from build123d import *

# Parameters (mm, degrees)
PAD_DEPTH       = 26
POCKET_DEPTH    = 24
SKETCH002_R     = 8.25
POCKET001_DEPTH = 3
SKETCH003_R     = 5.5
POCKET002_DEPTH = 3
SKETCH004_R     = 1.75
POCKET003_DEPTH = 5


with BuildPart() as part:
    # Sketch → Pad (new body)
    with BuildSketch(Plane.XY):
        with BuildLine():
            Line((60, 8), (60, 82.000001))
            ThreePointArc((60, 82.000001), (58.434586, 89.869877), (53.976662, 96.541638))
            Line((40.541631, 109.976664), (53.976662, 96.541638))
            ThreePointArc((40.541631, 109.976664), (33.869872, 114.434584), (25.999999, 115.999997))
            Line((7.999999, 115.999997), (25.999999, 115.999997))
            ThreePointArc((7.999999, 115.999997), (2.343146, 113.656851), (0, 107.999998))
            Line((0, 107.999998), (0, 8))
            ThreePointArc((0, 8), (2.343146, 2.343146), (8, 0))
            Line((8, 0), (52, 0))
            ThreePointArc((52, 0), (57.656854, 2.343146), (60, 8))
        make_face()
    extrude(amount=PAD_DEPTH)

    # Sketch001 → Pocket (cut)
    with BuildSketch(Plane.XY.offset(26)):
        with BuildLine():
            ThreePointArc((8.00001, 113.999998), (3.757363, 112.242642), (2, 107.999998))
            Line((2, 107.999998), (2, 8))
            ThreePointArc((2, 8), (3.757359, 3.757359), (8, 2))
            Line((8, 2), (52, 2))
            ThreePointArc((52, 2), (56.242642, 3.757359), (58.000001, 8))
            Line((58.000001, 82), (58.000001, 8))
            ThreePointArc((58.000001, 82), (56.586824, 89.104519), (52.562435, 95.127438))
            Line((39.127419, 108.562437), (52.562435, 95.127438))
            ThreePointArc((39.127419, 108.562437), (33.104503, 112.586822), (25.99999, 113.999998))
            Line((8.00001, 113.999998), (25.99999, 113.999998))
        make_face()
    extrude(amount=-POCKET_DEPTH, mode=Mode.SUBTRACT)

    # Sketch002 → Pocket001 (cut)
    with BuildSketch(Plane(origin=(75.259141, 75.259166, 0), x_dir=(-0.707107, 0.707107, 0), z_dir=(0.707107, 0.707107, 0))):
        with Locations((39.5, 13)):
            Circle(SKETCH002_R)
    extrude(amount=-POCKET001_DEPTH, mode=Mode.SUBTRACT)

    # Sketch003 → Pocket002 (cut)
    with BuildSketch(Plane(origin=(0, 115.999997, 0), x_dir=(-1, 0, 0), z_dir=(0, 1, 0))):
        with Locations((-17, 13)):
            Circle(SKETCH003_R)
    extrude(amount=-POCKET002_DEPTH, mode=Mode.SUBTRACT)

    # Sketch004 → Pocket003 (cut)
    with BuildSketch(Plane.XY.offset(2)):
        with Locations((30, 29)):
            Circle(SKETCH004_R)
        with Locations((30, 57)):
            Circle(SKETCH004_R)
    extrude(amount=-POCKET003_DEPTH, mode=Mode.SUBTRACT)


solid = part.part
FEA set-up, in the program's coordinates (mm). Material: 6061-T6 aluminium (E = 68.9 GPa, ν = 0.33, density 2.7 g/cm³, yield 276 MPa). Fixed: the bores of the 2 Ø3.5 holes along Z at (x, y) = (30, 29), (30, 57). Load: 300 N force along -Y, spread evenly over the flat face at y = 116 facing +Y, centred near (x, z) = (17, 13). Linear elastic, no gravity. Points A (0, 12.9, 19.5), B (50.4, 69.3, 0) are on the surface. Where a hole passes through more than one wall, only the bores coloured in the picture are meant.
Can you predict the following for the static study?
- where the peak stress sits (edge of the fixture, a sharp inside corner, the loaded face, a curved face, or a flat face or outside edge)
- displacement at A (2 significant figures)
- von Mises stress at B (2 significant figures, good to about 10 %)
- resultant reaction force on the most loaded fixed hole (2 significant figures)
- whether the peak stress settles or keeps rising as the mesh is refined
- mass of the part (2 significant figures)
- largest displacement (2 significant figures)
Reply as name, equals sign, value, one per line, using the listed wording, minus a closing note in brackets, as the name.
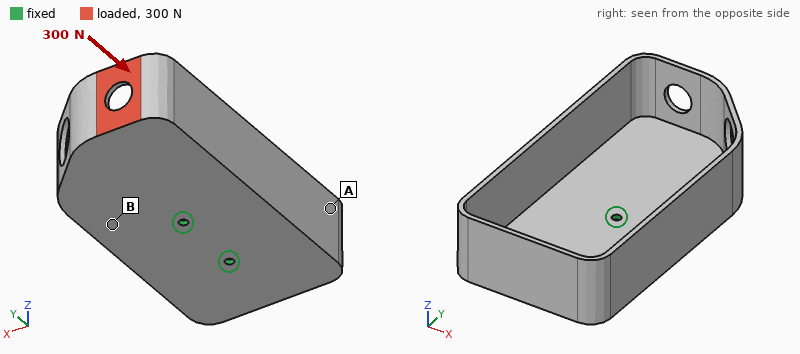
where the peak stress sits = edge of the fixture
displacement at A = 0.11 mm
von Mises stress at B = 12 MPa
resultant reaction force on the most loaded fixed hole = 230 N
whether the peak stress settles or keeps rising as the mesh is refined = keeps rising
mass of the part = 75 g
largest displacement = 0.31 mm
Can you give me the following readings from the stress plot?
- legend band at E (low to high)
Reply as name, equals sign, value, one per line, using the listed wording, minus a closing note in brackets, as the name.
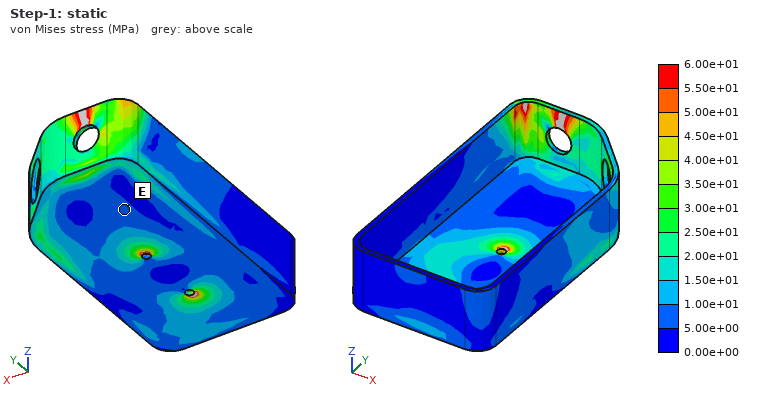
legend band at E = 5.00e+00 to 1.00e+01 MPa
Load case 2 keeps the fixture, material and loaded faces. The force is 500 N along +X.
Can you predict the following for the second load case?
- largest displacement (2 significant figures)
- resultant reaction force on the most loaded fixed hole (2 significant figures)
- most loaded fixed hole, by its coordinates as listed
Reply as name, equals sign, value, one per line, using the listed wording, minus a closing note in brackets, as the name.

largest displacement = 1.1 mm
resultant reaction force on the most loaded fixed hole = 1.5 kN
most loaded fixed hole, by its coordinates as listed = (30, 57)
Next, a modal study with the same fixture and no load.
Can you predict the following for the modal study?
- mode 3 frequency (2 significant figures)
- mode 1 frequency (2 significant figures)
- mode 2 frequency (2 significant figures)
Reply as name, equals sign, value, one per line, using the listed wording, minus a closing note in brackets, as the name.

mode 3 frequency = 880 Hz
mode 1 frequency = 490 Hz
mode 2 frequency = 570 Hz
